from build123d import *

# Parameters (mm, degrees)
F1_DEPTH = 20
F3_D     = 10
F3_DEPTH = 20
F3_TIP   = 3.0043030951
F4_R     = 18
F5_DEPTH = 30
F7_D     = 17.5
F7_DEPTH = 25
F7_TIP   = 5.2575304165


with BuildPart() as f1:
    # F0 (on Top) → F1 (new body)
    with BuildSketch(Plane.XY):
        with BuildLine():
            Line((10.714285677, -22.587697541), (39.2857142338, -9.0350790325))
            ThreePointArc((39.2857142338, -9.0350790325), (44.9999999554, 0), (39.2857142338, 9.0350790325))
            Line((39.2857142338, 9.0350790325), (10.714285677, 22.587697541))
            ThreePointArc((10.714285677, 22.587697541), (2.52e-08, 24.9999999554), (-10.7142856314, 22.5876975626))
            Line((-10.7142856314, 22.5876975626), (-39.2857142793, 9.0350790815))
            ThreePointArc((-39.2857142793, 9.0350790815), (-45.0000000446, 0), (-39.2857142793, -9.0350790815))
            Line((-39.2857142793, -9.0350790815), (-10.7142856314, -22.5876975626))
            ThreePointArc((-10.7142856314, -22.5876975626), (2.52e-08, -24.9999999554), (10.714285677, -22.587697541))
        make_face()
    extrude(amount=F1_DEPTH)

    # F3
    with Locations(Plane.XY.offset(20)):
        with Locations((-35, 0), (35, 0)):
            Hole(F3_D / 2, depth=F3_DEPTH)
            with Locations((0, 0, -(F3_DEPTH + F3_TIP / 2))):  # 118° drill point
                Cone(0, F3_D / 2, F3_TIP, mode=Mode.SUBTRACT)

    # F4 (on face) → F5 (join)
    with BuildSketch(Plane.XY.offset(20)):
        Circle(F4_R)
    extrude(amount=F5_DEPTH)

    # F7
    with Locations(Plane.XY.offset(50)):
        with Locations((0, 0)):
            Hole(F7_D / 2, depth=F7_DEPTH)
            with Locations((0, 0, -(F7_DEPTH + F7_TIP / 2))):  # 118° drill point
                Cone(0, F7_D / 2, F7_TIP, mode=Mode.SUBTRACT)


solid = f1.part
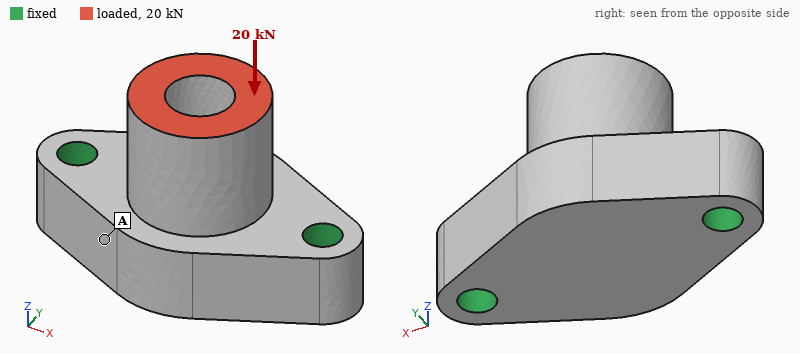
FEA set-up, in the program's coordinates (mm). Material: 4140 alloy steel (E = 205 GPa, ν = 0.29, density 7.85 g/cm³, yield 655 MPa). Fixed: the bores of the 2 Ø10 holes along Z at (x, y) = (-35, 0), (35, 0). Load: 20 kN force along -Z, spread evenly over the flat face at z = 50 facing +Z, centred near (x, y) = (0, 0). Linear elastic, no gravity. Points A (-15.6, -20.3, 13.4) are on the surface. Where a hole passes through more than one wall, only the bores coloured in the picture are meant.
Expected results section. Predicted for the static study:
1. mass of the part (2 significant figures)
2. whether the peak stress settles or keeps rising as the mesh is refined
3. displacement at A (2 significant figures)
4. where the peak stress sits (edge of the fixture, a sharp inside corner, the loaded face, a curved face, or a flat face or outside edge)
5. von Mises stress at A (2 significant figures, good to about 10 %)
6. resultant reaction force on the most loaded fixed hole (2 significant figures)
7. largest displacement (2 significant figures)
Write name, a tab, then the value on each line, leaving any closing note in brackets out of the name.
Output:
mass of the part	630 g
whether the peak stress settles or keeps rising as the mesh is refined	keeps rising
displacement at A	7.3 µm
where the peak stress sits	edge of the fixture
von Mises stress at A	18 MPa
resultant reaction force on the most loaded fixed hole	10 kN
largest displacement	12 µm
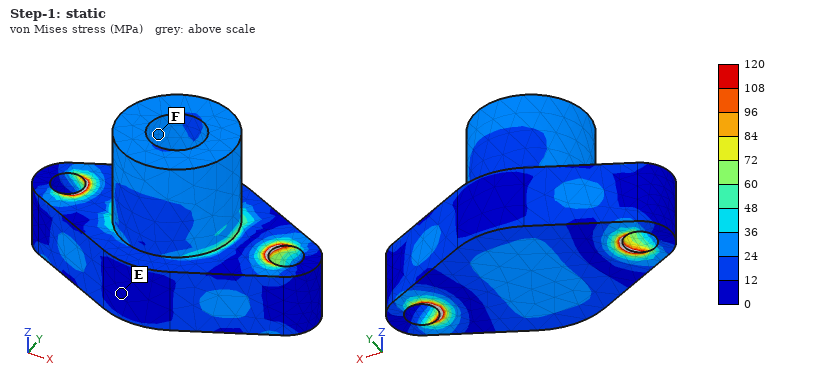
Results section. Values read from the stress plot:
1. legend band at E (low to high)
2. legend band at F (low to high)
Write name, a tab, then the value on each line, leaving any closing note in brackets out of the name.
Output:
legend band at E	0 to 12 MPa
legend band at F	24 to 36 MPa
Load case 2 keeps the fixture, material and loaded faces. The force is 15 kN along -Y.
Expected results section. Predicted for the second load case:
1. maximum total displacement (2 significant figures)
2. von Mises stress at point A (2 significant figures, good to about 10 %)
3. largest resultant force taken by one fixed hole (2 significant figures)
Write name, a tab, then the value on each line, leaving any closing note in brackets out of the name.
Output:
maximum total displacement	99 µm
von Mises stress at point A	83 MPa
largest resultant force taken by one fixed hole	7.5 kN
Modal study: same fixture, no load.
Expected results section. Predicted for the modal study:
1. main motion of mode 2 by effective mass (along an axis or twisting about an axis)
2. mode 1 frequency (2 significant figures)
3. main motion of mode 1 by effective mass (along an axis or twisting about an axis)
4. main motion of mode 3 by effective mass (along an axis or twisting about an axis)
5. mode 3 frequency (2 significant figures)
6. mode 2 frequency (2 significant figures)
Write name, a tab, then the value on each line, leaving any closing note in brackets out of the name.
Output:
main motion of mode 2 by effective mass	along Z
mode 1 frequency	6300 Hz
main motion of mode 1 by effective mass	along Y
main motion of mode 3 by effective mass	along X
mode 3 frequency	12 kHz
mode 2 frequency	11 kHz
